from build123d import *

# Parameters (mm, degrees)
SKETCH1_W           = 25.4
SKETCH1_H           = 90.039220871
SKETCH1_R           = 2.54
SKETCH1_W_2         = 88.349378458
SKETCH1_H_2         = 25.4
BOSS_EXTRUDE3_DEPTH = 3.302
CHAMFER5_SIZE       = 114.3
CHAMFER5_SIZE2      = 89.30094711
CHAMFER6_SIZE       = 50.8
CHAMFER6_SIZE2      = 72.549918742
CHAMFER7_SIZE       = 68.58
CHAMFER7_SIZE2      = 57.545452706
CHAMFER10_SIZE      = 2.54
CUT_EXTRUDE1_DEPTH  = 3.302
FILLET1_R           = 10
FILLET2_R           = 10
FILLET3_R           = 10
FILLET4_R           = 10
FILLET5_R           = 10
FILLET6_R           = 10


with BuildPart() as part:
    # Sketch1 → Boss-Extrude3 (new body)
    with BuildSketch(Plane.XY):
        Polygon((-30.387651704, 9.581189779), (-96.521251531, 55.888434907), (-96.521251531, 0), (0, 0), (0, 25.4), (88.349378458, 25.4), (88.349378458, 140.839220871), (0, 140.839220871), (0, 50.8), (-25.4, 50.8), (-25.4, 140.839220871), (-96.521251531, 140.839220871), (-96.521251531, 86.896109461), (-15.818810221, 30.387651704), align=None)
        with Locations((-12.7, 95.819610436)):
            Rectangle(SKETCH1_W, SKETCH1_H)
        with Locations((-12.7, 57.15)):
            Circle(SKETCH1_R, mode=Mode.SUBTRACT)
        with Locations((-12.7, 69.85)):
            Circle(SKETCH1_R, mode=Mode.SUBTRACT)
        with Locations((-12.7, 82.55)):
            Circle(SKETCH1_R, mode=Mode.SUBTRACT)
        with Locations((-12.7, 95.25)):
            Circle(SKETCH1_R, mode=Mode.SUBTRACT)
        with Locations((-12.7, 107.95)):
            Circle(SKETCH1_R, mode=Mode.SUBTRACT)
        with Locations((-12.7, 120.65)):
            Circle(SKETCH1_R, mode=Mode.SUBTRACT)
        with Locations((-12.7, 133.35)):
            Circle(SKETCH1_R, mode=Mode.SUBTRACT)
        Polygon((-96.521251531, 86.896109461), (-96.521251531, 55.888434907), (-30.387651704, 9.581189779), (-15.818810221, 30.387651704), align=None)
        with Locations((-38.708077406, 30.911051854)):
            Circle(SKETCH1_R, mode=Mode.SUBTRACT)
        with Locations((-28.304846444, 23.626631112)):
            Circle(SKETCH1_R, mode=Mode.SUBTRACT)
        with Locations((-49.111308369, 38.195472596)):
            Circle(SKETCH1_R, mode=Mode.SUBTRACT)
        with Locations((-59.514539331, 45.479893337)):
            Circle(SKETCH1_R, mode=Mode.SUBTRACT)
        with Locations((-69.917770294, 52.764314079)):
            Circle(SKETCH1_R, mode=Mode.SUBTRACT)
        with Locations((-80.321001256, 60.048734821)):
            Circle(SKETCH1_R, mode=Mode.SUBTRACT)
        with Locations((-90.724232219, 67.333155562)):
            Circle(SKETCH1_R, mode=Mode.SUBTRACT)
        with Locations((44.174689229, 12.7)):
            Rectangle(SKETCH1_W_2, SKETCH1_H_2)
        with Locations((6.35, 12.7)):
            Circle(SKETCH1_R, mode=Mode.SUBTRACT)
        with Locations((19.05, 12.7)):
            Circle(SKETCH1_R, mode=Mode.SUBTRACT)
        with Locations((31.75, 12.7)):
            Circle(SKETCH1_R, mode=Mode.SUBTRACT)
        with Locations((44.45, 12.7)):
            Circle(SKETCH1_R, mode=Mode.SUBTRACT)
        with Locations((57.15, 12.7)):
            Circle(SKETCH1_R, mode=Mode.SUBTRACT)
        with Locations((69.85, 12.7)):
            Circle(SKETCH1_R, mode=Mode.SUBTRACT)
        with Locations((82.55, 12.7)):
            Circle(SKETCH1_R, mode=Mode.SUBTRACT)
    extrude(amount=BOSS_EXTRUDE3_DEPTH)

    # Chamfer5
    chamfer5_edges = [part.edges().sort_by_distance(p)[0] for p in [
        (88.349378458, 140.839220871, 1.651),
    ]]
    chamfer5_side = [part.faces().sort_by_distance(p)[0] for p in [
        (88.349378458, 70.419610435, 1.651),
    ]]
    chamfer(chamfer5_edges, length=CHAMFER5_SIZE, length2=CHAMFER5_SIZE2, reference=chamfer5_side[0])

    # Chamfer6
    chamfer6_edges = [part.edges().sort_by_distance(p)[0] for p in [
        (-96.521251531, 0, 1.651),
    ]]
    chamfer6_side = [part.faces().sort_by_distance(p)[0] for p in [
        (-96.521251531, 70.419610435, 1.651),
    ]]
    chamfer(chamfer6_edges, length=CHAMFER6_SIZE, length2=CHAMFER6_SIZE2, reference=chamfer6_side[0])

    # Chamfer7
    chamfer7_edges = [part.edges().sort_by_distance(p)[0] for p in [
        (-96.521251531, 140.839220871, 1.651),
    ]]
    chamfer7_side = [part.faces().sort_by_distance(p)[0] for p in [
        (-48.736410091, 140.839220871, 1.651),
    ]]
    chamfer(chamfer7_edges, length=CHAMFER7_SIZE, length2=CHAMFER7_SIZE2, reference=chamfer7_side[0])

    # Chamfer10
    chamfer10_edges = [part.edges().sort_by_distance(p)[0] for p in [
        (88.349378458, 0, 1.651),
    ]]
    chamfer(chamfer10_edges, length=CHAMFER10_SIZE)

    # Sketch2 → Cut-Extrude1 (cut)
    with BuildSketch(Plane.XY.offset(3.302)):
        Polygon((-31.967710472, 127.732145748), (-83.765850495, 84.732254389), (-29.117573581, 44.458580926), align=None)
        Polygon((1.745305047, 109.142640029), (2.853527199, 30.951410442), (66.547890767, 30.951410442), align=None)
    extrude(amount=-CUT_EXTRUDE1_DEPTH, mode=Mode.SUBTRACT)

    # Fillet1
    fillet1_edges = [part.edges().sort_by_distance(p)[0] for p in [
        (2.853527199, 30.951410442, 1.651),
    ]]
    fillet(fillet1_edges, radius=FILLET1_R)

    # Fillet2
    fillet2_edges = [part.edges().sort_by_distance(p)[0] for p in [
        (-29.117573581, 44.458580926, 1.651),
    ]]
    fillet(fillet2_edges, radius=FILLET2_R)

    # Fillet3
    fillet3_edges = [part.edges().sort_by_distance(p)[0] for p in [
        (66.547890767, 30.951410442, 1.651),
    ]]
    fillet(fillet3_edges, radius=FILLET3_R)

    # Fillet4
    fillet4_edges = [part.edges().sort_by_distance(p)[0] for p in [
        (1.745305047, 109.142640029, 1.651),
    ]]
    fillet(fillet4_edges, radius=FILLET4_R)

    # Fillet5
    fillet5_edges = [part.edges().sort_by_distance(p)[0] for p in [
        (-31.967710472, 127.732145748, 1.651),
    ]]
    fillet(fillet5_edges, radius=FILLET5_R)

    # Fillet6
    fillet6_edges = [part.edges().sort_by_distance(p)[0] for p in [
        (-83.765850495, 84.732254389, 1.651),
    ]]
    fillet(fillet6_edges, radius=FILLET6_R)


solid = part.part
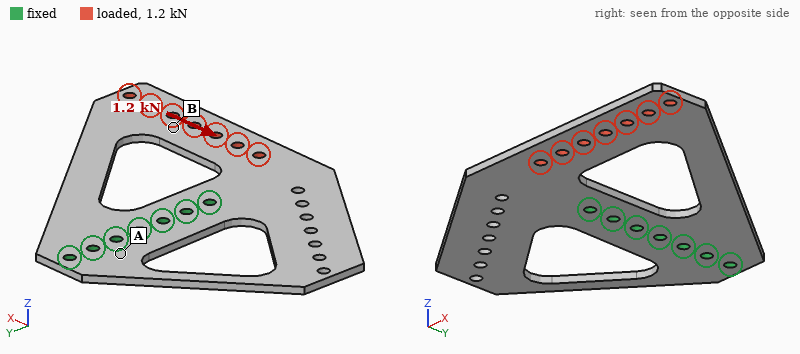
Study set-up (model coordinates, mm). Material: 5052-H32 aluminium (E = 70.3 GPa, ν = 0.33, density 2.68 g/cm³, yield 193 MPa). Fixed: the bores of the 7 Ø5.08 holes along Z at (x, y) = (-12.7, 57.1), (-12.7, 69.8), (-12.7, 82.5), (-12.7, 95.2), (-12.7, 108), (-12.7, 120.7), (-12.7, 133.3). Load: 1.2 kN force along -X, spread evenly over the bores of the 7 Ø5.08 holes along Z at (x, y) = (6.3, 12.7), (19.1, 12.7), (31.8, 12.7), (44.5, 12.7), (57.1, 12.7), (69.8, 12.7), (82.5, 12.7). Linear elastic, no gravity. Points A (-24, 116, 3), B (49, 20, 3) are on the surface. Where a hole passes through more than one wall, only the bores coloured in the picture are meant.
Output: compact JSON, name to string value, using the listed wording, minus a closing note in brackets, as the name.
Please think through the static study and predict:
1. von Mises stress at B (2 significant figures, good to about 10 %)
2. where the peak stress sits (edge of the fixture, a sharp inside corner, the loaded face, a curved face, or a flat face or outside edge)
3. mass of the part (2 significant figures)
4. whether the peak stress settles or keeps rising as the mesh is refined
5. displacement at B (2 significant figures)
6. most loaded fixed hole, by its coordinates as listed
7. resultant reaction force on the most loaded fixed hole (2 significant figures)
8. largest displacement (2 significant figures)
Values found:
{"von Mises stress at B": "9.9 MPa", "where the peak stress sits": "edge of the fixture", "mass of the part": "110 g", "whether the peak stress settles or keeps rising as the mesh is refined": "keeps rising", "displacement at B": "64 µm", "most loaded fixed hole, by its coordinates as listed": "(-12.7, 57.1)", "resultant reaction force on the most loaded fixed hole": "2.1 kN", "largest displacement": "82 µm"}
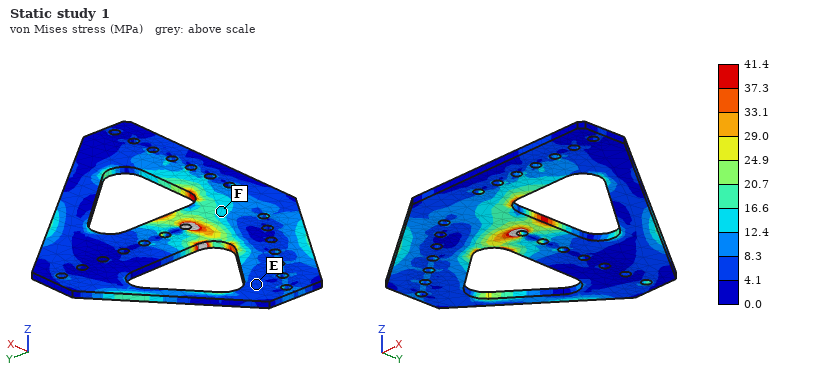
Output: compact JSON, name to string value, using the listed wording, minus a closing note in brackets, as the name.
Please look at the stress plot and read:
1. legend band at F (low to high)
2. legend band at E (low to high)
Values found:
{"legend band at F": "12.4 to 16.6 MPa", "legend band at E": "4.1 to 8.3 MPa"}
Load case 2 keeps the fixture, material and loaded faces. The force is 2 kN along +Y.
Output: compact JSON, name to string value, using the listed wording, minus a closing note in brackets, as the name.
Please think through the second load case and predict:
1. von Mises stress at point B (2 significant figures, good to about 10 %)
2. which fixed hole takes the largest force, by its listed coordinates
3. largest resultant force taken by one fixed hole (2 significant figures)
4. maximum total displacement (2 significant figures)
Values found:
{"von Mises stress at point B": "11 MPa", "which fixed hole takes the largest force, by its listed coordinates": "(-12.7, 57.1)", "largest resultant force taken by one fixed hole": "2.0 kN", "maximum total displacement": "0.12 mm"}
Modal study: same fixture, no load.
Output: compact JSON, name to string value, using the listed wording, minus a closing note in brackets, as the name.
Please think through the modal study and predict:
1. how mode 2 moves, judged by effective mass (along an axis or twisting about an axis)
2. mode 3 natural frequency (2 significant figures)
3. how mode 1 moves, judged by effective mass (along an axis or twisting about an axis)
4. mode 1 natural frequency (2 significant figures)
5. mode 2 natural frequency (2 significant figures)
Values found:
{"how mode 2 moves, judged by effective mass": "along Z", "mode 3 natural frequency": "690 Hz", "how mode 1 moves, judged by effective mass": "along Z", "mode 1 natural frequency": "230 Hz", "mode 2 natural frequency": "430 Hz"}
